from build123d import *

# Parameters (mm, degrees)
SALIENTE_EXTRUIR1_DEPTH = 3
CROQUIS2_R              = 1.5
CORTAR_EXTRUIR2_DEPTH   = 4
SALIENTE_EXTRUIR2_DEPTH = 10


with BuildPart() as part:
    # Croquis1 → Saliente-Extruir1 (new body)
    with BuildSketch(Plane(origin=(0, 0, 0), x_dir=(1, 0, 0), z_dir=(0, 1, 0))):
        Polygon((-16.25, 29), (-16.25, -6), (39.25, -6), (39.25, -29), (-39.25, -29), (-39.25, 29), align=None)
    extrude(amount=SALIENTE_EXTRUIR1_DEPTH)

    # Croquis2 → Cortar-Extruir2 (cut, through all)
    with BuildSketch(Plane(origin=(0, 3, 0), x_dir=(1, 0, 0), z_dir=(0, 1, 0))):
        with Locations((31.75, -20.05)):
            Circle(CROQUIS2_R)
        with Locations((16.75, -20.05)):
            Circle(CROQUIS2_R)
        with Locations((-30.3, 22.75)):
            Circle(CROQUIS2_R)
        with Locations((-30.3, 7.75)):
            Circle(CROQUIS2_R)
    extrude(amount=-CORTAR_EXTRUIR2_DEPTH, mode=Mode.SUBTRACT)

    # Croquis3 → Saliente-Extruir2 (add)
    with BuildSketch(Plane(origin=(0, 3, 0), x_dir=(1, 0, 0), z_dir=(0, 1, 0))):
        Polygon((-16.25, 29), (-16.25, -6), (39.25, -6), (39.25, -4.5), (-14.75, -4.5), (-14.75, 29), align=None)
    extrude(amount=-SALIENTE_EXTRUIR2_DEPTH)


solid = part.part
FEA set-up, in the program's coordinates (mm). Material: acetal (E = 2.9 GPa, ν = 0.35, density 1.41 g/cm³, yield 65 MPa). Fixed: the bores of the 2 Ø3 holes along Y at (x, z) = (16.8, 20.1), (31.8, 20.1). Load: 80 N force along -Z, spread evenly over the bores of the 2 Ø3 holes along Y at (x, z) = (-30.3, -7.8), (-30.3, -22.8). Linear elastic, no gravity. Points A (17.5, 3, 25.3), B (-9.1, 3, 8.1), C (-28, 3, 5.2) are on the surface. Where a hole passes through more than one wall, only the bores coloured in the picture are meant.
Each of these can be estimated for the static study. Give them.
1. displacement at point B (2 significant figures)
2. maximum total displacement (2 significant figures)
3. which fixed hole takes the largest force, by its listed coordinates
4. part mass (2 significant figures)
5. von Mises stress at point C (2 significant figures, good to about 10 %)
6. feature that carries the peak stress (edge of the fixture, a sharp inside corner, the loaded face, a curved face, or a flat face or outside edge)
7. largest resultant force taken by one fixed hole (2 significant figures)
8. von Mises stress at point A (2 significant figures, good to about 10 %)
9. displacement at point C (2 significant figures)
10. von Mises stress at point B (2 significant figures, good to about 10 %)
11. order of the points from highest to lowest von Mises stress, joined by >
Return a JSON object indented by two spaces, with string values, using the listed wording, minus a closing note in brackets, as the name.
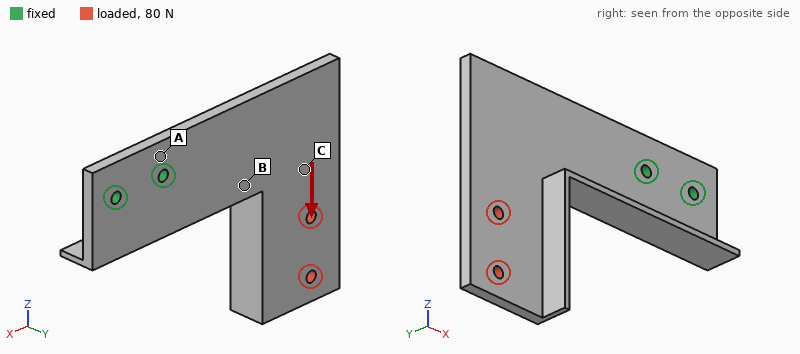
{
  "displacement at point B": "0.32 mm",
  "maximum total displacement": "1.1 mm",
  "which fixed hole takes the largest force, by its listed coordinates": "(16.8, 20.1)",
  "part mass": "13 g",
  "von Mises stress at point C": "1.7 MPa",
  "feature that carries the peak stress": "edge of the fixture",
  "largest resultant force taken by one fixed hole": "290 N",
  "von Mises stress at point A": "8.0 MPa",
  "displacement at point C": "0.64 mm",
  "von Mises stress at point B": "4.5 MPa",
  "order of the points from highest to lowest von Mises stress, joined by >": "A > B > C"
}
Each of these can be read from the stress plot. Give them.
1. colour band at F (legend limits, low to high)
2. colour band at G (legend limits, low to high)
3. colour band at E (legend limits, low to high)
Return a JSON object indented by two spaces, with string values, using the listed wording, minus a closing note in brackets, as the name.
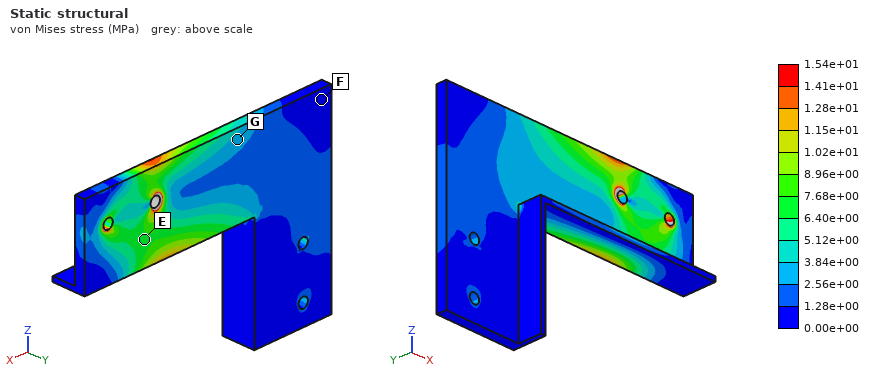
{
  "colour band at F": "0.00e+00 to 1.28e+00 MPa",
  "colour band at G": "2.56e+00 to 3.84e+00 MPa",
  "colour band at E": "6.40e+00 to 7.68e+00 MPa"
}
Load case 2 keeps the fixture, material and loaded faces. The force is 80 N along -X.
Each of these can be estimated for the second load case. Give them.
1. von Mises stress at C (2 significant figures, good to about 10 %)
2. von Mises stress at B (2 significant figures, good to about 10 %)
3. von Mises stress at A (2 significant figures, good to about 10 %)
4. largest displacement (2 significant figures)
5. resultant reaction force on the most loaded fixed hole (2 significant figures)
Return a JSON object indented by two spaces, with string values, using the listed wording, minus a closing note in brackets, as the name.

{
  "von Mises stress at C": "2.1 MPa",
  "von Mises stress at B": "8.2 MPa",
  "von Mises stress at A": "4.8 MPa",
  "largest displacement": "1.1 mm",
  "resultant reaction force on the most loaded fixed hole": "170 N"
}
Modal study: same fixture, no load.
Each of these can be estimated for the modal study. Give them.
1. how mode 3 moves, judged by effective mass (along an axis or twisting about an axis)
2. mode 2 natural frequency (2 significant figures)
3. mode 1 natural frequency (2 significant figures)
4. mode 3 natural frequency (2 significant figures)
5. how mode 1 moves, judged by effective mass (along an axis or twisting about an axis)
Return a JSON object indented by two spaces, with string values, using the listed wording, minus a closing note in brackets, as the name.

{
  "how mode 3 moves, judged by effective mass": "along Z",
  "mode 2 natural frequency": "330 Hz",
  "mode 1 natural frequency": "160 Hz",
  "mode 3 natural frequency": "670 Hz",
  "how mode 1 moves, judged by effective mass": "along Y"
}
